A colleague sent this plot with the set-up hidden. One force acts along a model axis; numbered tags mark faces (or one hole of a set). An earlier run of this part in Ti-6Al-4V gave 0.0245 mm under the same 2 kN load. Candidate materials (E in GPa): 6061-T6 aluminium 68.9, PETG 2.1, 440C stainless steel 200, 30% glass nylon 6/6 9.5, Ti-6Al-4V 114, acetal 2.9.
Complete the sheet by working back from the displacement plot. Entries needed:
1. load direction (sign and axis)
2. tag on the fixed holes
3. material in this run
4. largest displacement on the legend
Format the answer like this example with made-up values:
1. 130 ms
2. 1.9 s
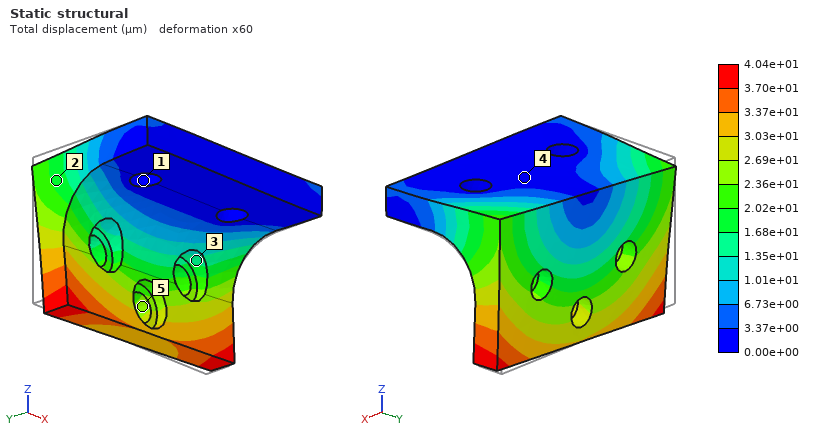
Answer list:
1. +X
2. 1
3. 6061-T6 aluminium
4. 4.04e+01 µm
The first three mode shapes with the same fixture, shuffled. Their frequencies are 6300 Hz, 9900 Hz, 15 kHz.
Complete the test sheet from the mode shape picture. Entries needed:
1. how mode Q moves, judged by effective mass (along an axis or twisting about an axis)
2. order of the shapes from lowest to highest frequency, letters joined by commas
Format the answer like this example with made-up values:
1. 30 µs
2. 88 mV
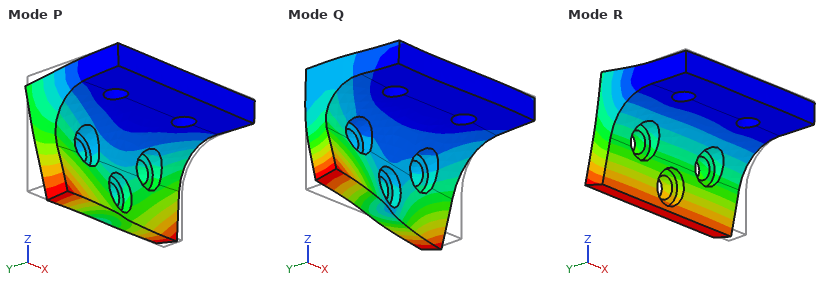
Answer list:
1. along X
2. R, P, Q
